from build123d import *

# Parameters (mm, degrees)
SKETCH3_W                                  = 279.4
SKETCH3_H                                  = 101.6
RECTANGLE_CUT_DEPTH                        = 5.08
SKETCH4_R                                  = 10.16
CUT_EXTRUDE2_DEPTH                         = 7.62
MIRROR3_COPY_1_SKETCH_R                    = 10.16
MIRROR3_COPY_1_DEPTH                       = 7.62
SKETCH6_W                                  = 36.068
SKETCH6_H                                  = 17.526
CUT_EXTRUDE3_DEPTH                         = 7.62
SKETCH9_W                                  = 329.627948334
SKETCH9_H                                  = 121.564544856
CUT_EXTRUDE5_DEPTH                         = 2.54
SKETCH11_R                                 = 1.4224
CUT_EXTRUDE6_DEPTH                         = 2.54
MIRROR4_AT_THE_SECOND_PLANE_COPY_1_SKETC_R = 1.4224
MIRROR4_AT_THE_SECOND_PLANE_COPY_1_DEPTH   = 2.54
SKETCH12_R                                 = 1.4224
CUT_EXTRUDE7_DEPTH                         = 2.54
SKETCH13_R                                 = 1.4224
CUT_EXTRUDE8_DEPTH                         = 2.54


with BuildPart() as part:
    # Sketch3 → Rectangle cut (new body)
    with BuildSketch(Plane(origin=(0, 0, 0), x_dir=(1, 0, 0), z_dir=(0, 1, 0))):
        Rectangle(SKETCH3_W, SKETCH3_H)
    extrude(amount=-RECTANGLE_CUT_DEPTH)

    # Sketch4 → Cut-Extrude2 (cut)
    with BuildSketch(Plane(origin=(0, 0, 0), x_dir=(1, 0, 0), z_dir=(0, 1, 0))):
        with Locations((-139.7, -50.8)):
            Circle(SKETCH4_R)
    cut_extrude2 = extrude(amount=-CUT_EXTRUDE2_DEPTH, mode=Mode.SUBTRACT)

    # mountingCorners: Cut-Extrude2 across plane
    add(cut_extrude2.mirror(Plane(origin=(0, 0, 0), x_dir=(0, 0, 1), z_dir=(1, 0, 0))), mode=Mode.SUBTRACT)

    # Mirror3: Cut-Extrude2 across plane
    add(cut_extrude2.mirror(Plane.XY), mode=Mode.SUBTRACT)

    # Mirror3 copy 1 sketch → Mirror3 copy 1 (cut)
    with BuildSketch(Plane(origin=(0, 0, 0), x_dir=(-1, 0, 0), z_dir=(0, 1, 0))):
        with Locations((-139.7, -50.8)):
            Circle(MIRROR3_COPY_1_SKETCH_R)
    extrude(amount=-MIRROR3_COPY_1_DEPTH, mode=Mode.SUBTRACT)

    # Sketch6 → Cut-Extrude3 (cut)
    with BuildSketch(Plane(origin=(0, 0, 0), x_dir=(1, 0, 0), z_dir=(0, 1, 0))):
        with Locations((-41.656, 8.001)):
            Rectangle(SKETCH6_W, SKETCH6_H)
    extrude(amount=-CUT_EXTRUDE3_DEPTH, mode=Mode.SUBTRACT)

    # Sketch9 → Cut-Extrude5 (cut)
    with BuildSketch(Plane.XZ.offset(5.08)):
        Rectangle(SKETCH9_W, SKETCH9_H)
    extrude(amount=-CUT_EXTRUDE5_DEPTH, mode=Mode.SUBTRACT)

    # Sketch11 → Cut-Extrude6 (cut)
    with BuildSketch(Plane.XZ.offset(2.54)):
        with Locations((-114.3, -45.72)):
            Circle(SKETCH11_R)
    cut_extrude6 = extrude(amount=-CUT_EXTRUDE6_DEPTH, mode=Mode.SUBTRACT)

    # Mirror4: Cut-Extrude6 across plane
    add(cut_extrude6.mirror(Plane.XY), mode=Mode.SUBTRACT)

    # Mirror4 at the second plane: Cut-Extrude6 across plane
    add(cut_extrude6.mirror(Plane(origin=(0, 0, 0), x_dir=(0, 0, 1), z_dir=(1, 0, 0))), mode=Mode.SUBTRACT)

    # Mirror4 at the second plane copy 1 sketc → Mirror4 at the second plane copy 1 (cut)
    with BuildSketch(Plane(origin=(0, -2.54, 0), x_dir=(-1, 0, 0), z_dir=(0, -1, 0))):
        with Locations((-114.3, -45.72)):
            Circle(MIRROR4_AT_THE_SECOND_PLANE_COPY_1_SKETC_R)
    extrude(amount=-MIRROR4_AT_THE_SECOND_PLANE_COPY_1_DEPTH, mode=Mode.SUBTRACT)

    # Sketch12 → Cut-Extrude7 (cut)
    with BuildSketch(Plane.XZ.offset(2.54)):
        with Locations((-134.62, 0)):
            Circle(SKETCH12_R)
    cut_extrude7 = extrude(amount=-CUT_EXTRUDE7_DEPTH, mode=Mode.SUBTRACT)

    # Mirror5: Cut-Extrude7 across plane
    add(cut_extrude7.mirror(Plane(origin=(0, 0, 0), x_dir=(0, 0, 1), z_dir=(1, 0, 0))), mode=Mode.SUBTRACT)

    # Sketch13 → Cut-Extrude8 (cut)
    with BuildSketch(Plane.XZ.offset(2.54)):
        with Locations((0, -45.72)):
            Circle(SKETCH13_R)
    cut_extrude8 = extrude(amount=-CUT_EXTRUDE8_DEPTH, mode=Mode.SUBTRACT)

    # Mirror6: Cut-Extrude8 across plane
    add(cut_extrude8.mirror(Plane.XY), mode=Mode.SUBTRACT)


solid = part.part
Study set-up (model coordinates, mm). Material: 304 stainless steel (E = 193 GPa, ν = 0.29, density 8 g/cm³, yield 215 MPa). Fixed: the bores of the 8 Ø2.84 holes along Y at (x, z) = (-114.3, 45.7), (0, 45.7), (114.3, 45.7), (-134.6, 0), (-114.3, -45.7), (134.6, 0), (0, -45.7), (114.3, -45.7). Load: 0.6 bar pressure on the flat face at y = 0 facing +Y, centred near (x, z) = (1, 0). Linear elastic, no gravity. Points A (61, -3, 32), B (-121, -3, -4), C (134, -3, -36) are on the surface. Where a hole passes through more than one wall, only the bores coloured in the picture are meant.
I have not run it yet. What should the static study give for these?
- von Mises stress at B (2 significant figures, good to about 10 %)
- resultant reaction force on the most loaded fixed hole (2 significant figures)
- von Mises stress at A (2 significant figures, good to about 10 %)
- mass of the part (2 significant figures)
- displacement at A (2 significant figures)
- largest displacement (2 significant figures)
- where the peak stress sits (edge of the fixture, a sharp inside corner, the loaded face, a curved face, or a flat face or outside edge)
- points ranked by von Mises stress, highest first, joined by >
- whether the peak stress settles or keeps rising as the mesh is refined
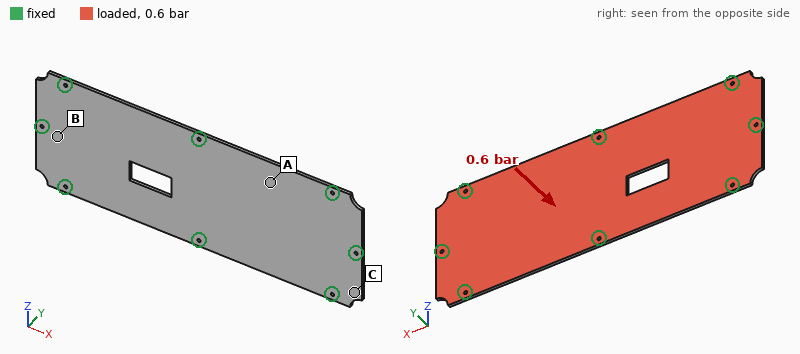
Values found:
20 MPa
350 N
33 MPa
560 g
0.15 mm
0.20 mm
edge of the fixture
A > B > C
keeps rising
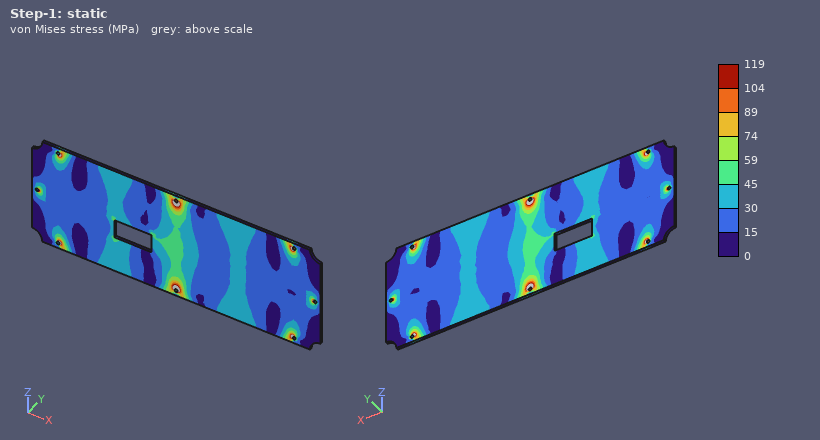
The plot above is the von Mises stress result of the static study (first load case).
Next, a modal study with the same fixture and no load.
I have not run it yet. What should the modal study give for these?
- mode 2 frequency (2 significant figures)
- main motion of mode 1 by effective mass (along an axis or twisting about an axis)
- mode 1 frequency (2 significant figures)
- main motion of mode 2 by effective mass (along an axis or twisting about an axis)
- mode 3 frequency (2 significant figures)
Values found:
760 Hz
twisting about Z
710 Hz
along Y
1100 Hz
